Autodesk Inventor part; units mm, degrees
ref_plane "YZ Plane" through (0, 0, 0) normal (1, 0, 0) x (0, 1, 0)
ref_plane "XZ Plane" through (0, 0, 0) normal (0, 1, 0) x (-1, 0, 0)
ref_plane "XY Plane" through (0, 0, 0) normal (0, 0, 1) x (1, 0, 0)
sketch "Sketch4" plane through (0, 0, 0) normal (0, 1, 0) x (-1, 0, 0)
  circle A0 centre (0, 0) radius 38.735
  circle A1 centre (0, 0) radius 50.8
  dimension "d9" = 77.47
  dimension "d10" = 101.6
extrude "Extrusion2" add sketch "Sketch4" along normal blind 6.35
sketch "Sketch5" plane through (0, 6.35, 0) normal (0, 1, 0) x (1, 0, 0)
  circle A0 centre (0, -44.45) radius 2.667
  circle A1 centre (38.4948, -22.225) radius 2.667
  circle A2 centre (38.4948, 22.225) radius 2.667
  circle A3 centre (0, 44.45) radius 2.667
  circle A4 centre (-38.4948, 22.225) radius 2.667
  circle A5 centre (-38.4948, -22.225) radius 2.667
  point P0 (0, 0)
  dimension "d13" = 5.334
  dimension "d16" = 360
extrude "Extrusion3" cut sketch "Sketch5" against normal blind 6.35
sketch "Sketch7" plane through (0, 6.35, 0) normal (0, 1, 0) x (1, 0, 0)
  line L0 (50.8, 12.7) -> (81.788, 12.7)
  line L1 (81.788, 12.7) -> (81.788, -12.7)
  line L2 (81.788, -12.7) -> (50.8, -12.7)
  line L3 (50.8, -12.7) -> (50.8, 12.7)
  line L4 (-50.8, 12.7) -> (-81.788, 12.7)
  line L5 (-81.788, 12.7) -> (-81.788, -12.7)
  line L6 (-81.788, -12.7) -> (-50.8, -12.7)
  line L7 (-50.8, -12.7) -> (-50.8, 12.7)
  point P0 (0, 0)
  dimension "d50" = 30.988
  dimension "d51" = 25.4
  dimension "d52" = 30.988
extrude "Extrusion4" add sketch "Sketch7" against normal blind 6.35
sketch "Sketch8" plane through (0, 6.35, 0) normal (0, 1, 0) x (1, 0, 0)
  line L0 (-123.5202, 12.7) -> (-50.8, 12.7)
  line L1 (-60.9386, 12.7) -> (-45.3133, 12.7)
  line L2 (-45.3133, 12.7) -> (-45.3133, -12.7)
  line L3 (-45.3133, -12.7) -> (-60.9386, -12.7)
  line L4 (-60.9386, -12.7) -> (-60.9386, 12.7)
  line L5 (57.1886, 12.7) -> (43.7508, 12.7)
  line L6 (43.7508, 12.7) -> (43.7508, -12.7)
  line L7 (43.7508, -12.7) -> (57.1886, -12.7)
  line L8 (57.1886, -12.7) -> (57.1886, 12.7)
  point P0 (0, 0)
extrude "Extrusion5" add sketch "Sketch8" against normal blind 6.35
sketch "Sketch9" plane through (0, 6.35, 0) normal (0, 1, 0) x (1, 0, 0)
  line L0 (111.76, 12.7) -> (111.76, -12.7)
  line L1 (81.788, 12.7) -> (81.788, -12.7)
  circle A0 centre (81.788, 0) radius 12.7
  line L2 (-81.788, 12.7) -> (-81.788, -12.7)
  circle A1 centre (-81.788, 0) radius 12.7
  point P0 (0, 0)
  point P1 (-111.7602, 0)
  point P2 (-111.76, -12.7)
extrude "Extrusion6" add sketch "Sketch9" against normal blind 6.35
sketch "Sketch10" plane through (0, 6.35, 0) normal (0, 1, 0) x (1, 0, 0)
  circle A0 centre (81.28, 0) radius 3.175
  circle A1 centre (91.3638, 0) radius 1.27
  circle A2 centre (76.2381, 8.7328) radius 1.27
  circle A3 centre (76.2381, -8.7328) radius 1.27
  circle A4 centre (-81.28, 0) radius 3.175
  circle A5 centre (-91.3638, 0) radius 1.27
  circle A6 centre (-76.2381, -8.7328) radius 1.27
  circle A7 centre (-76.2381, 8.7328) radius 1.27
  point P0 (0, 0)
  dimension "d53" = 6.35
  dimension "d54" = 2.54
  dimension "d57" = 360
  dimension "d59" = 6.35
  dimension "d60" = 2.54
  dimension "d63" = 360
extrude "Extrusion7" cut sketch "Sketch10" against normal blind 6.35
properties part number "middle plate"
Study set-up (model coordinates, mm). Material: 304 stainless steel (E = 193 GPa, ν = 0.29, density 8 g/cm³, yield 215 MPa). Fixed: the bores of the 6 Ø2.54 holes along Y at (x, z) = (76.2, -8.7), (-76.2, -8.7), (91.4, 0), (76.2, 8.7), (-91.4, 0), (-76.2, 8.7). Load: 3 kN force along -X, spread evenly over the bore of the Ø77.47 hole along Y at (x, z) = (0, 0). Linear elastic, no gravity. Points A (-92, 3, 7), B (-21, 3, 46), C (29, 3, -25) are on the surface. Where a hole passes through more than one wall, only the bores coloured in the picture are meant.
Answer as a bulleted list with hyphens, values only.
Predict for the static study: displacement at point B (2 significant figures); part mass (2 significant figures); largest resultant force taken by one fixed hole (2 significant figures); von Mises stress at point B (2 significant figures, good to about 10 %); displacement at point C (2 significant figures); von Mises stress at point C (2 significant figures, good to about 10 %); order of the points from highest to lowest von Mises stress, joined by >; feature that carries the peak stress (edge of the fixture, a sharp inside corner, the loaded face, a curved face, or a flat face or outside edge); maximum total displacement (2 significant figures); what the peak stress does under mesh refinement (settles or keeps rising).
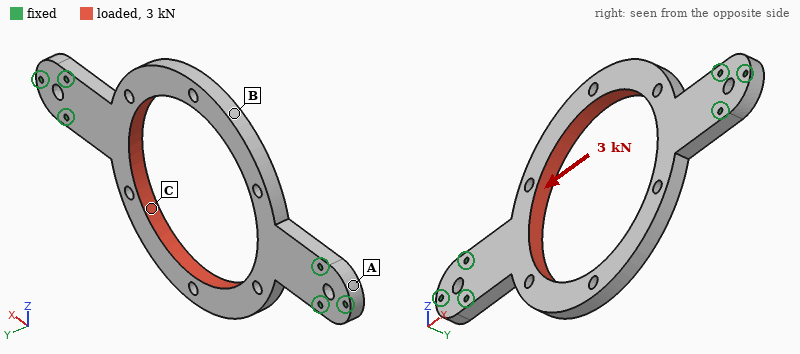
- 12 µm
- 270 g
- 720 N
- 16 MPa
- 10 µm
- 26 MPa
- C > B > A
- a sharp inside corner
- 13 µm
- keeps rising
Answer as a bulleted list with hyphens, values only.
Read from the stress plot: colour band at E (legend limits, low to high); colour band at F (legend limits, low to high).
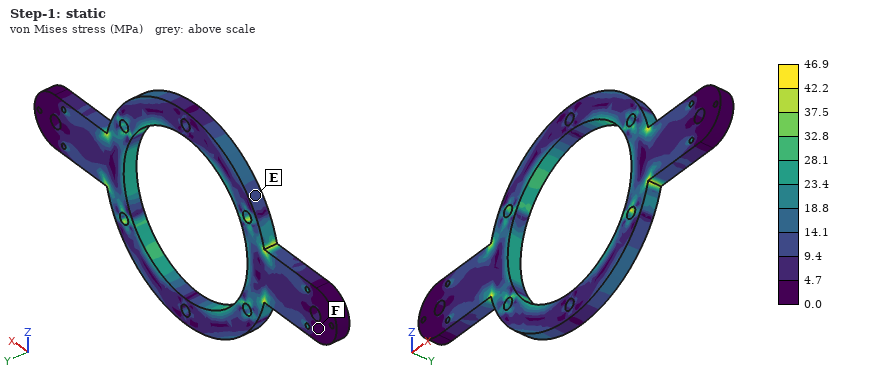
- 9.4 to 14.1 MPa
- 0.0 to 4.7 MPa
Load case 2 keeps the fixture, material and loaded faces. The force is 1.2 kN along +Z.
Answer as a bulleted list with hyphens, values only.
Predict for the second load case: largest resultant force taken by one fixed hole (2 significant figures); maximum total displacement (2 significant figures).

- 730 N
- 4.7 µm
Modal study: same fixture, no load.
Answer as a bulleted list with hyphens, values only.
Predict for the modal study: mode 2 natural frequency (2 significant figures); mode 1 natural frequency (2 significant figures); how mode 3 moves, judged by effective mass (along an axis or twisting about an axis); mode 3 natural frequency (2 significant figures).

- 1000 Hz
- 970 Hz
- twisting about Z
- 2600 Hz
